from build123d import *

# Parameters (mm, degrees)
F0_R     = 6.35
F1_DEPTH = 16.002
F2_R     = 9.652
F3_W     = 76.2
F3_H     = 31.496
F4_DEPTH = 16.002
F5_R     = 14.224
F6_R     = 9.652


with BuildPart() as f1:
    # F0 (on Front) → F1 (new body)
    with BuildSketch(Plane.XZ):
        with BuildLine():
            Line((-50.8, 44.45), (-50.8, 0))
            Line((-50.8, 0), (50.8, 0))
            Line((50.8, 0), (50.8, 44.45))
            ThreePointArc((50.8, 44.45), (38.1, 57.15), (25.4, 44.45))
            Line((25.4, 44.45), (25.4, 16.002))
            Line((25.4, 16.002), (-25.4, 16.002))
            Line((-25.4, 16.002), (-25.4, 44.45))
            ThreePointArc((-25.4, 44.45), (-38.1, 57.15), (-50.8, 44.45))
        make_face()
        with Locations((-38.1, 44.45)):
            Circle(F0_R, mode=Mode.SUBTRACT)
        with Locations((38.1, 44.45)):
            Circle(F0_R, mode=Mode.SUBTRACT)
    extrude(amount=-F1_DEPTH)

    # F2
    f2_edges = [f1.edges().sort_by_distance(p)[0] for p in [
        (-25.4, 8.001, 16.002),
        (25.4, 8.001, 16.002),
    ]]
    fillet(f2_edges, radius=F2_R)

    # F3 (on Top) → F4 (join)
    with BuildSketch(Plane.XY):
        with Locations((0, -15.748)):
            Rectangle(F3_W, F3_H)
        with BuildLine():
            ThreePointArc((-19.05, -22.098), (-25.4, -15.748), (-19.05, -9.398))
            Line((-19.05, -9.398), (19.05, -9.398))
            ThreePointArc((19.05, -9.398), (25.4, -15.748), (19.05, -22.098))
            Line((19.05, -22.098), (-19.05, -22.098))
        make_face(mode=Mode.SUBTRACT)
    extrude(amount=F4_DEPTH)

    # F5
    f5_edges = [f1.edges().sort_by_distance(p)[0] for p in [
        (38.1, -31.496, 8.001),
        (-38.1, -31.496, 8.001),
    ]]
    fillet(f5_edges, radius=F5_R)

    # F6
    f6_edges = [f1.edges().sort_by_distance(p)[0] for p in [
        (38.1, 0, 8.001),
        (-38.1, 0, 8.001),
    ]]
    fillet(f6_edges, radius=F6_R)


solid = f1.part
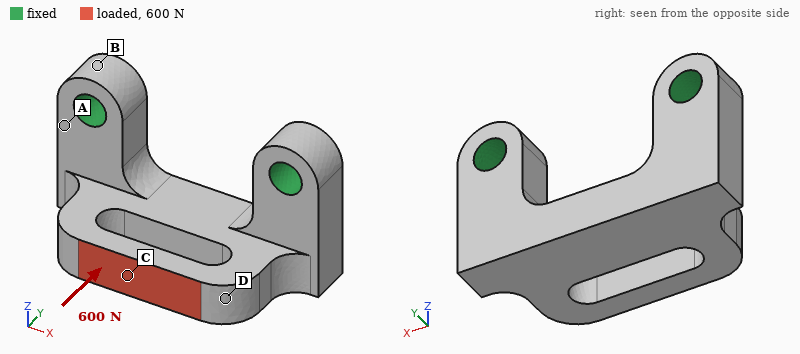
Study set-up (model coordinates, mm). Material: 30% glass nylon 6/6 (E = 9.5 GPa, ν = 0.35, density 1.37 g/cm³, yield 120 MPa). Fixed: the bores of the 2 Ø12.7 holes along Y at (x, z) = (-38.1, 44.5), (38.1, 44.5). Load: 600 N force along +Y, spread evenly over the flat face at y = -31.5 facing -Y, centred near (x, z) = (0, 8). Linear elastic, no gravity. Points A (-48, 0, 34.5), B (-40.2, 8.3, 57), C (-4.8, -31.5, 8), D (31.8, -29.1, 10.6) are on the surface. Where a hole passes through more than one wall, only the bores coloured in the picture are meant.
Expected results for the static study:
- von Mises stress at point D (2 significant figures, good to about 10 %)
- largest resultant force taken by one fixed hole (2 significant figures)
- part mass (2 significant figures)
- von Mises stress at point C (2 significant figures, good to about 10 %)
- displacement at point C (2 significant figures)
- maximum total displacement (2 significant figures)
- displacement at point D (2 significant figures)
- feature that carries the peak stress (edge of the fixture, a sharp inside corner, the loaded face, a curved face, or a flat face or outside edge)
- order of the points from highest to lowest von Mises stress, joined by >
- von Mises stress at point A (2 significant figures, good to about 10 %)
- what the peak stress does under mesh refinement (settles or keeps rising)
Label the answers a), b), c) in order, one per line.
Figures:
a) 2.9 MPa
b) 300 N
c) 110 g
d) 7.8 MPa
e) 0.12 mm
f) 0.14 mm
g) 0.088 mm
h) edge of the fixture
i) C > A > D > B
j) 5.4 MPa
k) keeps rising
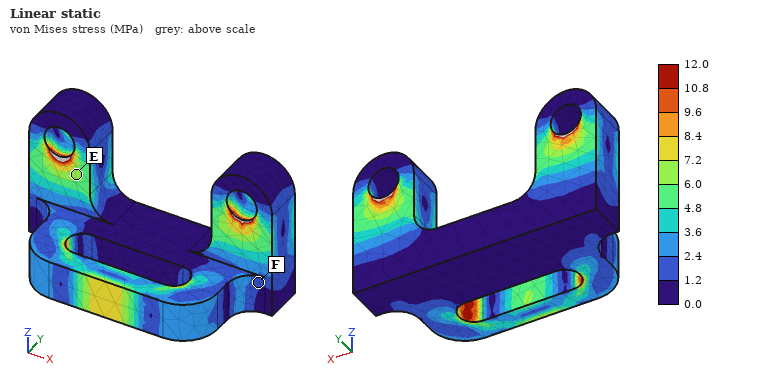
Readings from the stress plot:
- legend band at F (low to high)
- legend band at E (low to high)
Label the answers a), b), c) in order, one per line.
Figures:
a) 1.2 to 2.4 MPa
b) 6.0 to 7.2 MPa
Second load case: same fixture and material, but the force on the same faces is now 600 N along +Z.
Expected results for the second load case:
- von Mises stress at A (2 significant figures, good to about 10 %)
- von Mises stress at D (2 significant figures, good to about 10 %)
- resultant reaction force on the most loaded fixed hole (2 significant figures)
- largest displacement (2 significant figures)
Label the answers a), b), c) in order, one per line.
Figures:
a) 8.5 MPa
b) 4.1 MPa
c) 330 N
d) 0.36 mm
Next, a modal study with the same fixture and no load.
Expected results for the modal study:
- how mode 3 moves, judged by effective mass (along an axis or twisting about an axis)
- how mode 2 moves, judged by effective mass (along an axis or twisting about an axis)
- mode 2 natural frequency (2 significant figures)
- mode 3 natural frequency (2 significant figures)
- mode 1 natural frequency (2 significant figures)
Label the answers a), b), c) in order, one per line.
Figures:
a) along Y
b) along X
c) 2700 Hz
d) 3400 Hz
e) 1500 Hz
